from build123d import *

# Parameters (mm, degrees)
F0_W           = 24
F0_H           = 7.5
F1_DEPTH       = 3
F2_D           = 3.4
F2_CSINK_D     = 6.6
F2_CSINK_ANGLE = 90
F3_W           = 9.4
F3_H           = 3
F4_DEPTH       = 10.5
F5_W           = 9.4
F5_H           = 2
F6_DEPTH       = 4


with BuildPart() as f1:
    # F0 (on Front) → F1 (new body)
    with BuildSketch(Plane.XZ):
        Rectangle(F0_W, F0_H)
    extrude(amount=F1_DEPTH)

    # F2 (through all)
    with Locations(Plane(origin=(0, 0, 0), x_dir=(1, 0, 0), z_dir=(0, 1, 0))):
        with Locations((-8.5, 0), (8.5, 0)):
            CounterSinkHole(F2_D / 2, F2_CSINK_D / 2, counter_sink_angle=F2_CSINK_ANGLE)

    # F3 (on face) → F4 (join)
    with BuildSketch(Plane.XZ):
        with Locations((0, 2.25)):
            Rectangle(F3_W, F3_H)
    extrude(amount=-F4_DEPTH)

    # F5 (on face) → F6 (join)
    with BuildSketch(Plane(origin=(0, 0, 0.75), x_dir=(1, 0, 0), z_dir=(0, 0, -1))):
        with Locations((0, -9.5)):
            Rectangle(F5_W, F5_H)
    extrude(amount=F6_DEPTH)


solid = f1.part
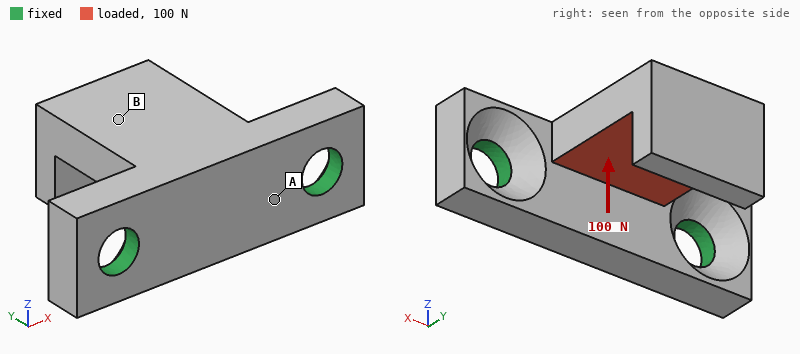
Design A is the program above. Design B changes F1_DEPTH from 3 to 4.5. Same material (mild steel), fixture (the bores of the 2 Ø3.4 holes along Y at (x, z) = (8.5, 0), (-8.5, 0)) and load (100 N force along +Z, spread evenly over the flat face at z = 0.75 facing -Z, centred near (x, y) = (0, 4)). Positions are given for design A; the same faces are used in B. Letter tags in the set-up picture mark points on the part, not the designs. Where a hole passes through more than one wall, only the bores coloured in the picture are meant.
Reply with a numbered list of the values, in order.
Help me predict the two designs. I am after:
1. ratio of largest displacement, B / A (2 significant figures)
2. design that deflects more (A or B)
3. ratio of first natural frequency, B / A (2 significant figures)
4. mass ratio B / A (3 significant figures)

1. 0.64
2. A
3. 1.2
4. 1.30
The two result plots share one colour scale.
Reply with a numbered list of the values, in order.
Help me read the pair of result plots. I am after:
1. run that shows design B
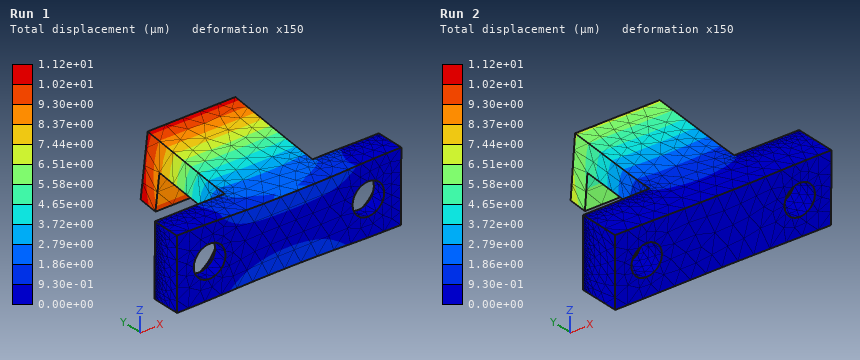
1. Run 2
